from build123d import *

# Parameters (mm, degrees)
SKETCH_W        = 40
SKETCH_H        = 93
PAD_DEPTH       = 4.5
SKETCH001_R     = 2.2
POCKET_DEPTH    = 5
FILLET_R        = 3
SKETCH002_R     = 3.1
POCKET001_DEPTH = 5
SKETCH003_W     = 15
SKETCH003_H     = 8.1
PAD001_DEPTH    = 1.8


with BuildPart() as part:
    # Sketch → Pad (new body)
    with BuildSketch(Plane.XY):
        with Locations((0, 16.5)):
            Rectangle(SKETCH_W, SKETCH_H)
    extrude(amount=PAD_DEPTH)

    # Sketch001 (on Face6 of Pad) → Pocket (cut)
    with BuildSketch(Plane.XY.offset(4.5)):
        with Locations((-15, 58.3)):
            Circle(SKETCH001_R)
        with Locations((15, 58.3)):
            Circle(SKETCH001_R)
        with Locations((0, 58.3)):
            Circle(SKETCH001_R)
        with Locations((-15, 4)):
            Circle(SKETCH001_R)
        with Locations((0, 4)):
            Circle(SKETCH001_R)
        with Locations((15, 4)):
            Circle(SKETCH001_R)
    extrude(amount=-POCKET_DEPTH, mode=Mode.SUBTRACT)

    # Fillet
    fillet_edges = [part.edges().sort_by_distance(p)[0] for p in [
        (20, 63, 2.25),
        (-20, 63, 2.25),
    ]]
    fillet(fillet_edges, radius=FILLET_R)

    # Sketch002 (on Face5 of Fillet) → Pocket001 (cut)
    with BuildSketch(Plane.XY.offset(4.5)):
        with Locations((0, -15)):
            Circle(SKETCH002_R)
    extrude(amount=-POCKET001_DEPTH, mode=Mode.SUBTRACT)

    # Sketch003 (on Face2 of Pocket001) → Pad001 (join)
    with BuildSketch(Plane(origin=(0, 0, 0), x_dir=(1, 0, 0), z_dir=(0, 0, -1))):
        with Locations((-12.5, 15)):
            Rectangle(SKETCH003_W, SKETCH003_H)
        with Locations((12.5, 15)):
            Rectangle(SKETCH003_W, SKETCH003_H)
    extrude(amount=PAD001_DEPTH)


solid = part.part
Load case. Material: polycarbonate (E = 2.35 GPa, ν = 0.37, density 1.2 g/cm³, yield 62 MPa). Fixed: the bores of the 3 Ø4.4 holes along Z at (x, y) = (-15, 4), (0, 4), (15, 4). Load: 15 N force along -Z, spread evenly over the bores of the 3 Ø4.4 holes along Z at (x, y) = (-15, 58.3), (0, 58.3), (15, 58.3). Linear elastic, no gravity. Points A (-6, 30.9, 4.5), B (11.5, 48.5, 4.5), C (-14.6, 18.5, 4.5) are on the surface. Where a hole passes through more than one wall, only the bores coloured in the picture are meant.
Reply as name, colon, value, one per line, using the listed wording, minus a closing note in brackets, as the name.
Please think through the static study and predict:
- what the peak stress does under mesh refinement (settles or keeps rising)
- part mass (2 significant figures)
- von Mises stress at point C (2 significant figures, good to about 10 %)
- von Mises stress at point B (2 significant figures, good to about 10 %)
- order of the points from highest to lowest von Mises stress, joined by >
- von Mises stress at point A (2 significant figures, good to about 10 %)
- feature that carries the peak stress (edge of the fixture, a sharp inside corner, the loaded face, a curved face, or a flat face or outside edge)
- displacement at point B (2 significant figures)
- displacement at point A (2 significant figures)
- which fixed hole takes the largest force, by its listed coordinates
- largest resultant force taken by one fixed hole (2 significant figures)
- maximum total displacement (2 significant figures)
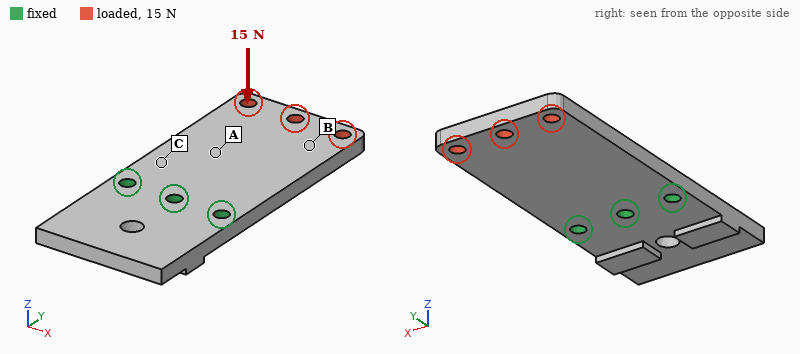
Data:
what the peak stress does under mesh refinement: keeps rising
part mass: 20 g
von Mises stress at point C: 4.3 MPa
von Mises stress at point B: 1.2 MPa
order of the points from highest to lowest von Mises stress, joined by >: C > A > B
von Mises stress at point A: 2.8 MPa
feature that carries the peak stress: edge of the fixture
displacement at point B: 0.74 mm
displacement at point A: 0.31 mm
which fixed hole takes the largest force, by its listed coordinates: (0, 4)
largest resultant force taken by one fixed hole: 14 N
maximum total displacement: 1.2 mm
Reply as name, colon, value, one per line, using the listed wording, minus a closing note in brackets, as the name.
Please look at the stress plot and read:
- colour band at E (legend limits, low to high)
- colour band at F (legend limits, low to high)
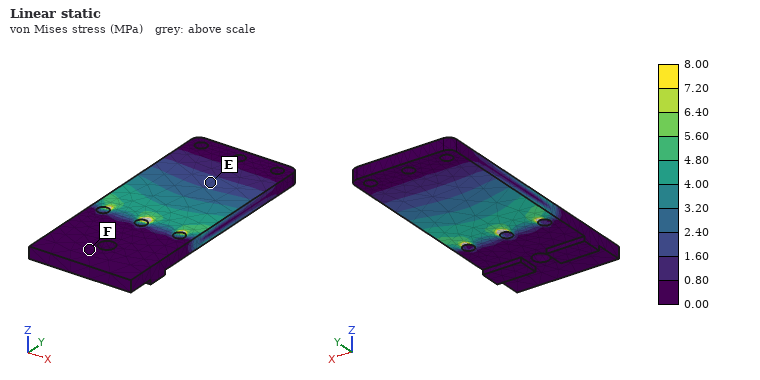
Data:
colour band at E: 1.60 to 2.40 MPa
colour band at F: 0.00 to 0.80 MPa
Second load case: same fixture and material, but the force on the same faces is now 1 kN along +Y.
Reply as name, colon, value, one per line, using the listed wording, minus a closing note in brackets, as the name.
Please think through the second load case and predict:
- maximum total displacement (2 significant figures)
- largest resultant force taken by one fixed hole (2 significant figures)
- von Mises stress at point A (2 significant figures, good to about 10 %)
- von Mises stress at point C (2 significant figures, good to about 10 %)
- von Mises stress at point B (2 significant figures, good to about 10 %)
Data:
maximum total displacement: 0.16 mm
largest resultant force taken by one fixed hole: 340 N
von Mises stress at point A: 5.5 MPa
von Mises stress at point C: 5.6 MPa
von Mises stress at point B: 5.4 MPa
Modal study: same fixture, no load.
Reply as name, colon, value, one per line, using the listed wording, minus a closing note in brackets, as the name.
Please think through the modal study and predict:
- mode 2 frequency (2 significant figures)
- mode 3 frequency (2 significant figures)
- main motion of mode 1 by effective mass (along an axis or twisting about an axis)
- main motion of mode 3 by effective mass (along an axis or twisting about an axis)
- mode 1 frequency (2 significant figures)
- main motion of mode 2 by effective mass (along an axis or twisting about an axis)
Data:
mode 2 frequency: 930 Hz
mode 3 frequency: 980 Hz
main motion of mode 1 by effective mass: along Z
main motion of mode 3 by effective mass: twisting about Y
mode 1 frequency: 320 Hz
main motion of mode 2 by effective mass: along Z
